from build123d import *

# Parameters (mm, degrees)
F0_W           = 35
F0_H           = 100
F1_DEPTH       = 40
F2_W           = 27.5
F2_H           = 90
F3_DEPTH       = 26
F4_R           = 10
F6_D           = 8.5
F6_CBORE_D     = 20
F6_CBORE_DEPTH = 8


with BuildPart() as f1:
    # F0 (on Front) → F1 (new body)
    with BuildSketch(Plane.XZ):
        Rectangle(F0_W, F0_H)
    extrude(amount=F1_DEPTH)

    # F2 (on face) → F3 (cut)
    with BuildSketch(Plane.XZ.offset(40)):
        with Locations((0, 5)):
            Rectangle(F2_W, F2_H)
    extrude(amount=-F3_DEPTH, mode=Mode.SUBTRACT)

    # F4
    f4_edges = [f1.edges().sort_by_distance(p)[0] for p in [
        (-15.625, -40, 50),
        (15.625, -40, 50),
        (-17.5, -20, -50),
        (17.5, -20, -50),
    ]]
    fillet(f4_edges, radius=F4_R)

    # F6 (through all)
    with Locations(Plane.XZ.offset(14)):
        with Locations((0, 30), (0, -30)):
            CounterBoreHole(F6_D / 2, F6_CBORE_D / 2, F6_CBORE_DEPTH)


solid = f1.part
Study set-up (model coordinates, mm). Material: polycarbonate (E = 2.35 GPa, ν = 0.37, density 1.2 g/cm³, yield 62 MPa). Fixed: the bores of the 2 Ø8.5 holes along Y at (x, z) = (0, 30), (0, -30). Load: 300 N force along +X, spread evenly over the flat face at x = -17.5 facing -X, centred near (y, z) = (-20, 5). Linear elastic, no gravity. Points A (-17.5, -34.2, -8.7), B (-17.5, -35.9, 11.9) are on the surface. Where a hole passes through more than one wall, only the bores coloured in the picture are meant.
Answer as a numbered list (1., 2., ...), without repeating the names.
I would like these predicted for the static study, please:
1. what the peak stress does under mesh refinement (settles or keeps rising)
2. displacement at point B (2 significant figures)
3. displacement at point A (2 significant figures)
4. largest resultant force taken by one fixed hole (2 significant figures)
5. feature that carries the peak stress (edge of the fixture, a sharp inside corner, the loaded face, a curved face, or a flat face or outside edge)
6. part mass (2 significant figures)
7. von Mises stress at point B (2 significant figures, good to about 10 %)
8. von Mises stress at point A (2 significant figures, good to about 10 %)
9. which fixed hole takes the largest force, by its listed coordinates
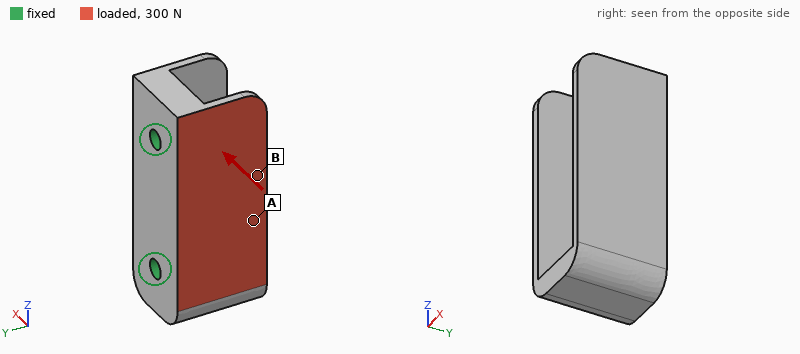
1. keeps rising
2. 0.60 mm
3. 0.45 mm
4. 170 N
5. edge of the fixture
6. 82 g
7. 1.0 MPa
8. 2.9 MPa
9. (0, 30)
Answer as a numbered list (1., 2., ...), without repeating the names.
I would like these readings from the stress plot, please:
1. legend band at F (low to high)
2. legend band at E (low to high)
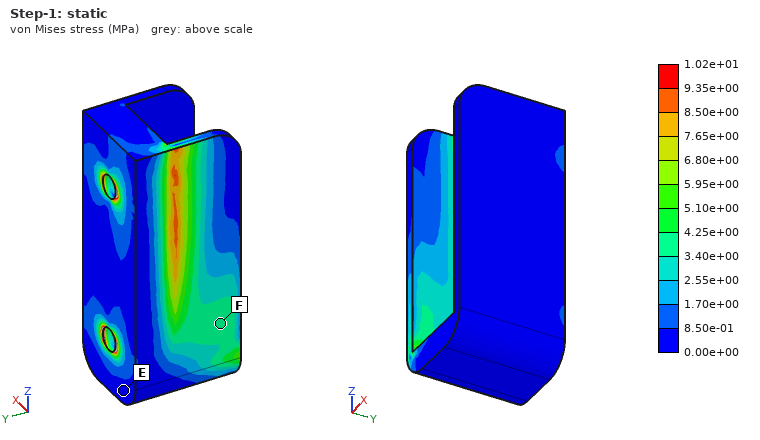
1. 3.40e+00 to 4.25e+00 MPa
2. 0.00e+00 to 8.50e-01 MPa
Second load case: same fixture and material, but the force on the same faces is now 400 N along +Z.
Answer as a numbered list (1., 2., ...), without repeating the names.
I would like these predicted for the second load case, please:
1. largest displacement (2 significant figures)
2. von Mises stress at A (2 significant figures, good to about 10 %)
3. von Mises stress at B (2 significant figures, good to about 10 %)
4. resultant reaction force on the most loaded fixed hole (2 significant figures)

1. 68 µm
2. 0.40 MPa
3. 0.63 MPa
4. 250 N
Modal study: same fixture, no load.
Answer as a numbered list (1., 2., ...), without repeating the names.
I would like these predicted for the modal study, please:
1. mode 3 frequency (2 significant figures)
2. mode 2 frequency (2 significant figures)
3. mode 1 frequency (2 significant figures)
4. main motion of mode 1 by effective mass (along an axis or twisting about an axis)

1. 1200 Hz
2. 1200 Hz
3. 850 Hz
4. along X
